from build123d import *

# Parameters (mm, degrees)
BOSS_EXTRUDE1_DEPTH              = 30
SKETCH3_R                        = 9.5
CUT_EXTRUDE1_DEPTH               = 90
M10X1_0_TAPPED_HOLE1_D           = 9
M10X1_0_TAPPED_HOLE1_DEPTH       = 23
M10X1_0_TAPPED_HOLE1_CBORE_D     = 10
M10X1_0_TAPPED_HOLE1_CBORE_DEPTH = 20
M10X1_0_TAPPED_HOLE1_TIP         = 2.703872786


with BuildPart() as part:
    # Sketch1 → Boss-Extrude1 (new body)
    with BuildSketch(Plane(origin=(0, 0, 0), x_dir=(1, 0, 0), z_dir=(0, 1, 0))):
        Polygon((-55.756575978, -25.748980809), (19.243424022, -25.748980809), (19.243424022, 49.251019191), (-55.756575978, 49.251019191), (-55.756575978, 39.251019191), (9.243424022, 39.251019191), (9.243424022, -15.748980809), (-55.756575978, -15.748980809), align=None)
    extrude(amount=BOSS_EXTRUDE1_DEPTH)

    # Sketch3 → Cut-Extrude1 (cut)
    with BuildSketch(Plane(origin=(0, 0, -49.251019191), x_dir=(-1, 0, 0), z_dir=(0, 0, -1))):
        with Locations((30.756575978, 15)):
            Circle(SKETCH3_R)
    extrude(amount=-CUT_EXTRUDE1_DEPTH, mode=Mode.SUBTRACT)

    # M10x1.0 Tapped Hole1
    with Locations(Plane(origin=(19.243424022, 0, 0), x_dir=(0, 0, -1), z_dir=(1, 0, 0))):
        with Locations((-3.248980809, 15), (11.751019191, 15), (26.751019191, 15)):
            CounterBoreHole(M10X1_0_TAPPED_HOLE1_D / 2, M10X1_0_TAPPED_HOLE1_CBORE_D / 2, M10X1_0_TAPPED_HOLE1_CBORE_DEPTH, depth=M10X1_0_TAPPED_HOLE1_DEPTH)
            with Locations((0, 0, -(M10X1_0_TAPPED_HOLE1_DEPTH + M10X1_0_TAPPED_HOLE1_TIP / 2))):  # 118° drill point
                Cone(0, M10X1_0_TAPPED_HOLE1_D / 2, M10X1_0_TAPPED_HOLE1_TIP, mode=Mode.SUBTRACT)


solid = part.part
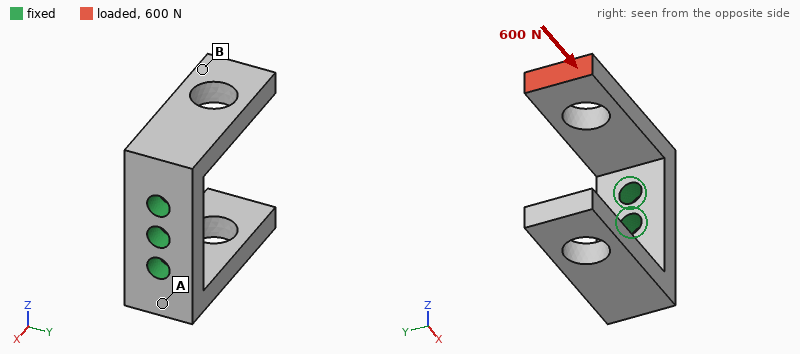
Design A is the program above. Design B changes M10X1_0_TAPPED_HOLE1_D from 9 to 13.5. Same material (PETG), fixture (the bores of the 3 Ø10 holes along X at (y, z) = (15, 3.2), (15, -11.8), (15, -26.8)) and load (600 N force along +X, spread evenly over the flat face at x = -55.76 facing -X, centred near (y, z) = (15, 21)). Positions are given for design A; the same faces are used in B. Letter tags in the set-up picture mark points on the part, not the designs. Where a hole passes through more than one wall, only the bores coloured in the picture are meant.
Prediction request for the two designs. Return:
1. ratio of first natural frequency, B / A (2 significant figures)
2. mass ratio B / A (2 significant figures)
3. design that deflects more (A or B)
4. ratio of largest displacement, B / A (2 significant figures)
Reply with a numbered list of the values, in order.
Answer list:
1. 1.0
2. 0.96
3. A
4. 0.77
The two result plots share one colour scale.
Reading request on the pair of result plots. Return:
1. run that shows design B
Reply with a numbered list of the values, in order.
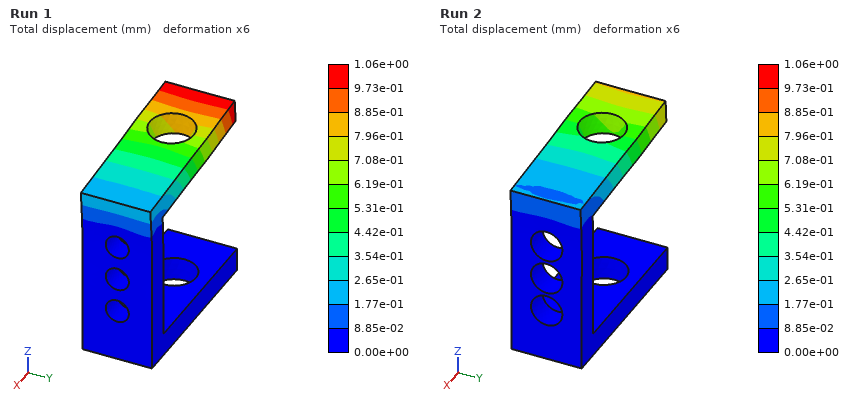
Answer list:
1. Run 2
